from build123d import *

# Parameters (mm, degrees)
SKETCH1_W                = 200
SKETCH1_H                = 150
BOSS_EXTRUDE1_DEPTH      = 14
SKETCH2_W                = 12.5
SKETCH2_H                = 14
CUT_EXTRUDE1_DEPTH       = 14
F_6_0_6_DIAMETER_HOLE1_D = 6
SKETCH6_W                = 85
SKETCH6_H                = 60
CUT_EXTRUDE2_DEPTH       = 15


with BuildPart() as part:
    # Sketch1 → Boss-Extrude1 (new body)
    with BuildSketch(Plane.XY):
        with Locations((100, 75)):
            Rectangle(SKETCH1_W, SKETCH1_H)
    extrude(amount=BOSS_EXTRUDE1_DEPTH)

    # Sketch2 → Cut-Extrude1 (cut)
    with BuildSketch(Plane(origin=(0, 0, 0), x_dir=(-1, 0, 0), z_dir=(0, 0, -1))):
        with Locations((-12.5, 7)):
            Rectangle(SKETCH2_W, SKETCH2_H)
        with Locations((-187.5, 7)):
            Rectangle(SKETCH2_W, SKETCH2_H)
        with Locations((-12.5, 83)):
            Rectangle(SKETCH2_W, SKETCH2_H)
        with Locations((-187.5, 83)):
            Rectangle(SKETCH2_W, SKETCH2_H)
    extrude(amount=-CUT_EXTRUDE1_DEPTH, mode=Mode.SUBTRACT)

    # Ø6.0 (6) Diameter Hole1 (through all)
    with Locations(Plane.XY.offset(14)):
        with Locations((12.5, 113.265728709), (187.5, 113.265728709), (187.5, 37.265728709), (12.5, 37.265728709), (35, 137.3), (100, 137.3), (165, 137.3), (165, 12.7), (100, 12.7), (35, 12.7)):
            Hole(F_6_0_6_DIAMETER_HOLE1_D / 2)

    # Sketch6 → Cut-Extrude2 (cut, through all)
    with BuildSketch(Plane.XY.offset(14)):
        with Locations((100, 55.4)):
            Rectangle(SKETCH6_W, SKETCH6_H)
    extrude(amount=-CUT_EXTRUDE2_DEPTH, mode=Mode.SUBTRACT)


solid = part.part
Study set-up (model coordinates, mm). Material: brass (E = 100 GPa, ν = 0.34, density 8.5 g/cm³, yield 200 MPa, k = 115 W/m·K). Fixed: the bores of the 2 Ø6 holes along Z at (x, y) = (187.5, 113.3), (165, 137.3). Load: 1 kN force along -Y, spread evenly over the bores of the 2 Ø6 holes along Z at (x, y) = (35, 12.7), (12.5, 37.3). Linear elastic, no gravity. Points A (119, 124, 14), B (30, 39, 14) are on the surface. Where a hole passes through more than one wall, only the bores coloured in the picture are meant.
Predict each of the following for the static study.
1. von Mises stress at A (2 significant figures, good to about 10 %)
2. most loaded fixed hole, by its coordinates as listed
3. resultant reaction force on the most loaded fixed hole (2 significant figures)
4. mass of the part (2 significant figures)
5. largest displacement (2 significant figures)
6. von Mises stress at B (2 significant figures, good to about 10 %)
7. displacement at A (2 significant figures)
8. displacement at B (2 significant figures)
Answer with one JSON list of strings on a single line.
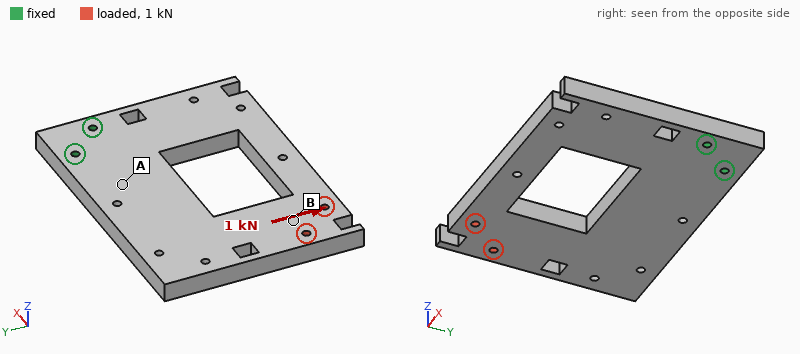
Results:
["3.3 MPa", "(165, 137.3)", "4.5 kN", "2.8 kg", "56 µm", "1.8 MPa", "12 µm", "46 µm"]
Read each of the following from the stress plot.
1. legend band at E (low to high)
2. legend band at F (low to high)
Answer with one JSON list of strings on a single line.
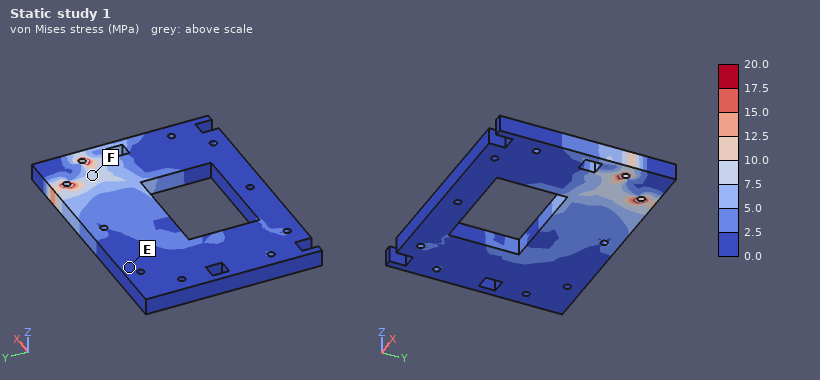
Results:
["0.0 to 2.5 MPa", "7.5 to 10.0 MPa"]
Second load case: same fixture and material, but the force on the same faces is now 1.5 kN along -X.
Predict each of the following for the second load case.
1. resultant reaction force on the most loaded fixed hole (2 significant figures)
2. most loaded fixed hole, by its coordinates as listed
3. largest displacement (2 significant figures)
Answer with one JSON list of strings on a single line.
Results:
["4.6 kN", "(187.5, 113.3)", "60 µm"]
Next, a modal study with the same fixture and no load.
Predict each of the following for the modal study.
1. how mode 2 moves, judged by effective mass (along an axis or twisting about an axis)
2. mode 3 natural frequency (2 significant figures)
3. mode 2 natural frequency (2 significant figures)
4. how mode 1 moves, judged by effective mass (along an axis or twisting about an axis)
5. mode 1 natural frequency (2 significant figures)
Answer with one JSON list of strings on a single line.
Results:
["twisting about X", "620 Hz", "400 Hz", "along Z", "180 Hz"]
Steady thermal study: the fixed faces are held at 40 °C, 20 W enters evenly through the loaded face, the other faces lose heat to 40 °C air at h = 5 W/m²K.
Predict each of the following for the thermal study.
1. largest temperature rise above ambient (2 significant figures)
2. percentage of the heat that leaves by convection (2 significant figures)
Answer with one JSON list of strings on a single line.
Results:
["28 K", "20 %"]
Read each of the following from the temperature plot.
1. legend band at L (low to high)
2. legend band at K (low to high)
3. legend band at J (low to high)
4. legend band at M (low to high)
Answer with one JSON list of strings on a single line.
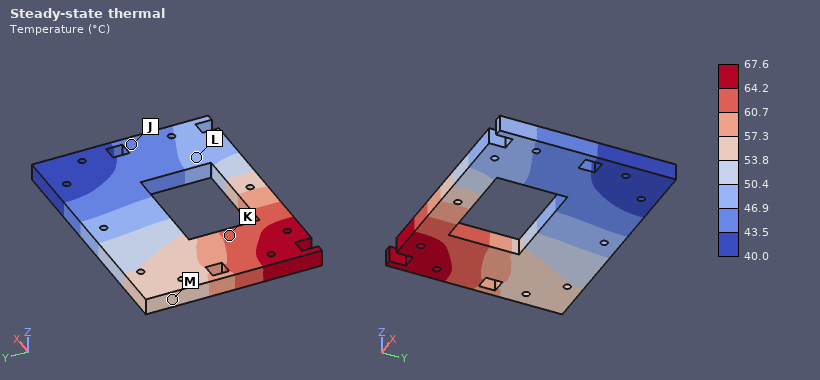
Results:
["46.9 to 50.4 °C", "60.7 to 64.2 °C", "43.5 to 46.9 °C", "53.8 to 57.3 °C"]
